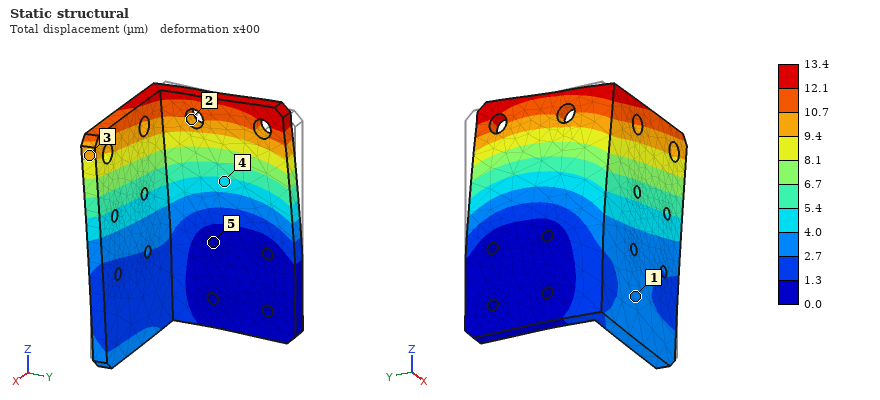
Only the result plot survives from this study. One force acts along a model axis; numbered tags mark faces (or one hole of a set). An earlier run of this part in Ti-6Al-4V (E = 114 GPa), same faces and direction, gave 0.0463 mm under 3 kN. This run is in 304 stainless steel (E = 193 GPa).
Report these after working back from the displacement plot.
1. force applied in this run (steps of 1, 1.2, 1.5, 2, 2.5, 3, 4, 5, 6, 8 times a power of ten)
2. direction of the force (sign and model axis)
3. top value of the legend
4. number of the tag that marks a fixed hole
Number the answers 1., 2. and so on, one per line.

1. 1.5 kN
2. -Y
3. 13.4 µm
4. 5
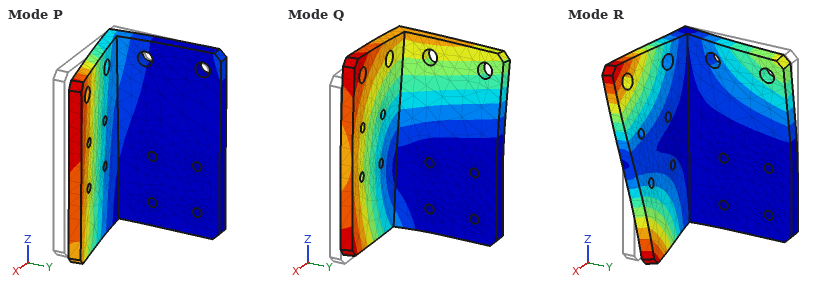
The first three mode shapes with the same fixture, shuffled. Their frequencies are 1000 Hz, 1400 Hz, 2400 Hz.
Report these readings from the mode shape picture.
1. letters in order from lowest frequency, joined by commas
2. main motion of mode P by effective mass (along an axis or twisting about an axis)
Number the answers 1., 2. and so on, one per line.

1. P, Q, R
2. along Y
